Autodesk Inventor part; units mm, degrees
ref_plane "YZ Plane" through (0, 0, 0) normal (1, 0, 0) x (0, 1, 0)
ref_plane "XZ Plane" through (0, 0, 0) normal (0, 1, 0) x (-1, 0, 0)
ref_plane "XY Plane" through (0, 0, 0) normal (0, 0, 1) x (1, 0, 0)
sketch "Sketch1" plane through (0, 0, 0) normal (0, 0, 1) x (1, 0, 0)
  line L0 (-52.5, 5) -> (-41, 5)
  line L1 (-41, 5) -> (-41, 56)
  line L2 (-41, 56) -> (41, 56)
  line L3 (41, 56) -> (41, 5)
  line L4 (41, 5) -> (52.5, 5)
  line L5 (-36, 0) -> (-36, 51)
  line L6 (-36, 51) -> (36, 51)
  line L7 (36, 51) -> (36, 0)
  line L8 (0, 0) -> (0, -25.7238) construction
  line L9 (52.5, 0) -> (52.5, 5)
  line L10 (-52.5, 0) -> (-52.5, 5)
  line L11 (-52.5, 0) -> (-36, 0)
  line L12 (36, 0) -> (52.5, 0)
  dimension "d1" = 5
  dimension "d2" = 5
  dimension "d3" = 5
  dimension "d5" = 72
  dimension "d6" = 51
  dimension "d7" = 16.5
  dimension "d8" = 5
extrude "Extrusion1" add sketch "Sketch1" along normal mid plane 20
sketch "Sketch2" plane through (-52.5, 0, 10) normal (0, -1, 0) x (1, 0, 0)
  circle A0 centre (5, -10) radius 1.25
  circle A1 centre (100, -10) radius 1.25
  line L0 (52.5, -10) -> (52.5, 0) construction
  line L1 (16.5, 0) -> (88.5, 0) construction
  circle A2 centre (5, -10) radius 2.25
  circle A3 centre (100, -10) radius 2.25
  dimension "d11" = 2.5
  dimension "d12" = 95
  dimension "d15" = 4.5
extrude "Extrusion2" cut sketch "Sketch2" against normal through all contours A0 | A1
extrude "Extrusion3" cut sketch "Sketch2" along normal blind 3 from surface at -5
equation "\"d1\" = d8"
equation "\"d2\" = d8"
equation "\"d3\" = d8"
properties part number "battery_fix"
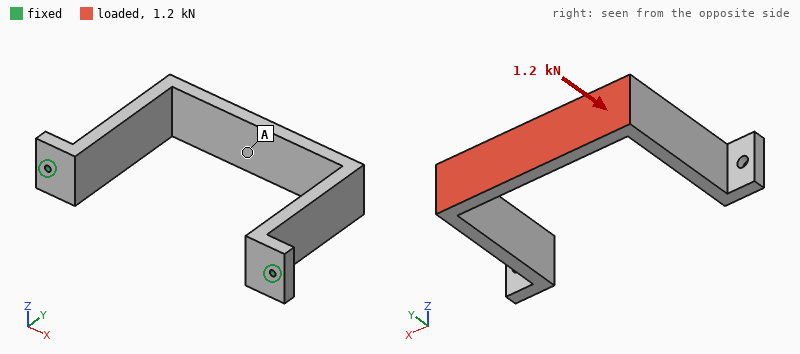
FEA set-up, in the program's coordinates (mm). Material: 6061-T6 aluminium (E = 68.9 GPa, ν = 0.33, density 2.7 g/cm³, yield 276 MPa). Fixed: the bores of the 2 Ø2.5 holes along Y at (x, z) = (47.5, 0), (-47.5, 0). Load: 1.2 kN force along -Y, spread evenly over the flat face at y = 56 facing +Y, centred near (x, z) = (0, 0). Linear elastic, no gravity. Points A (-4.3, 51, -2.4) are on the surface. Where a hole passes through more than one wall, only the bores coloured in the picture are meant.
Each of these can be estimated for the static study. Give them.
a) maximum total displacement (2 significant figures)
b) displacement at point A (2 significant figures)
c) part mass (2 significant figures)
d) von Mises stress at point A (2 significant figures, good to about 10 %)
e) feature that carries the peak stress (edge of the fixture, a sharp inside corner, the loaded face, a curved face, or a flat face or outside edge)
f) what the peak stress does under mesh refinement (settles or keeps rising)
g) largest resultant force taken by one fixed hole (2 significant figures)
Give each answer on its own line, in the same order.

0.19 mm
0.18 mm
56 g
54 MPa
edge of the fixture
keeps rising
630 N
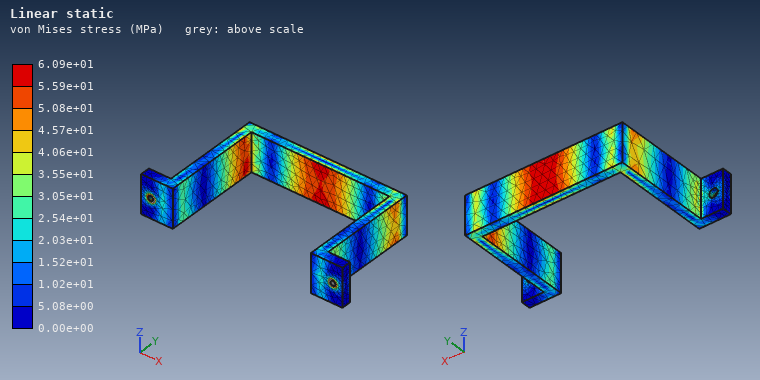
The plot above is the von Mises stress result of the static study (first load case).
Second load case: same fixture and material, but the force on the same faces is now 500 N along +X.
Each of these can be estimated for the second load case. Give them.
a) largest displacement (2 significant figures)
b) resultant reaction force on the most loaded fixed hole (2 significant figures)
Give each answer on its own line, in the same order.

0.52 mm
330 N
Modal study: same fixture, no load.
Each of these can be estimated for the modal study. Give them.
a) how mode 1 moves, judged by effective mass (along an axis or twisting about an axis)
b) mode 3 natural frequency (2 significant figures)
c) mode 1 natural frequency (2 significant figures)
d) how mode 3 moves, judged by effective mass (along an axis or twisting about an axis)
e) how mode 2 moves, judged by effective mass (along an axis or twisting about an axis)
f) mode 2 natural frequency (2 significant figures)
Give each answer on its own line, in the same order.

along Z
1300 Hz
560 Hz
twisting about Y
along X
870 Hz
